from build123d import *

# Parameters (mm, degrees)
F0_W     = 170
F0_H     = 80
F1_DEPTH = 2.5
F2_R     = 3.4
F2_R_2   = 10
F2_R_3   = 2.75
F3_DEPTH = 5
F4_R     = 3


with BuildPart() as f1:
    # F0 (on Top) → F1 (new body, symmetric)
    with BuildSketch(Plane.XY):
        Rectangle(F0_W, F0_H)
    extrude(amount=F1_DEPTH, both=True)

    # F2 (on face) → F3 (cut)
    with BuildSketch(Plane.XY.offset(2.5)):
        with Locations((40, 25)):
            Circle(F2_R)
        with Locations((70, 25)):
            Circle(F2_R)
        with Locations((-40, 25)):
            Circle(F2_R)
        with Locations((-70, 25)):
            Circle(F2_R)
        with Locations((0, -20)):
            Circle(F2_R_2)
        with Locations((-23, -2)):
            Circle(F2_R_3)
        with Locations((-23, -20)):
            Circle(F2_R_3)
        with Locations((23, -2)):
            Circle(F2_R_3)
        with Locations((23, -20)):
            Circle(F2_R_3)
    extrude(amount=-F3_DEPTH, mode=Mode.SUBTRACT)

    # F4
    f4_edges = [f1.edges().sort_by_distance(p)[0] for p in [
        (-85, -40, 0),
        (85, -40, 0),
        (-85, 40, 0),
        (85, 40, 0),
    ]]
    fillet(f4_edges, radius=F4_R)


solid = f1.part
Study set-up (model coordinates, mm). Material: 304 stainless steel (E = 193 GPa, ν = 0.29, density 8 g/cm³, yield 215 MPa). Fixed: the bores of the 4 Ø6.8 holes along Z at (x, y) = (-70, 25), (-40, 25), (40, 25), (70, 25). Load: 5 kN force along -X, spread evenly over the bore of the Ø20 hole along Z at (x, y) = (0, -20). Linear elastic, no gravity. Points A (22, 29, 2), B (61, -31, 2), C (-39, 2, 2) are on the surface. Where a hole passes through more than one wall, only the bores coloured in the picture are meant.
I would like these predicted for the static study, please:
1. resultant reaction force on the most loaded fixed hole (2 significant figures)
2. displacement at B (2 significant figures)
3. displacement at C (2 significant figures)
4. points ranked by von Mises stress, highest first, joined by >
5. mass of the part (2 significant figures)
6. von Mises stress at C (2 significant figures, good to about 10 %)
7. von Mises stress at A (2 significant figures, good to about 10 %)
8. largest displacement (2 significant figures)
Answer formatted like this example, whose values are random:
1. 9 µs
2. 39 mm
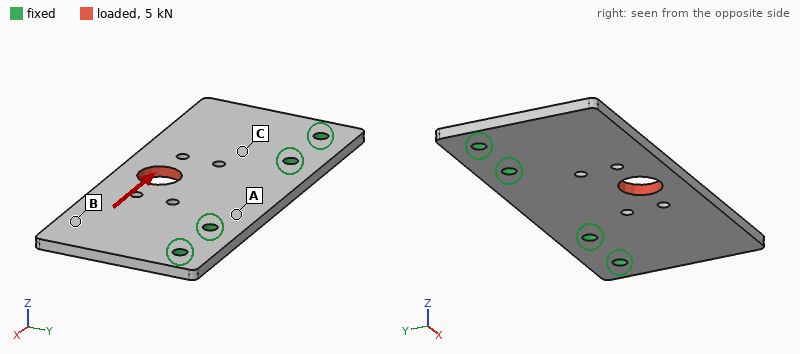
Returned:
1. 1.7 kN
2. 5.3 µm
3. 2.6 µm
4. C > A > B
5. 520 g
6. 11 MPa
7. 6.9 MPa
8. 8.1 µm
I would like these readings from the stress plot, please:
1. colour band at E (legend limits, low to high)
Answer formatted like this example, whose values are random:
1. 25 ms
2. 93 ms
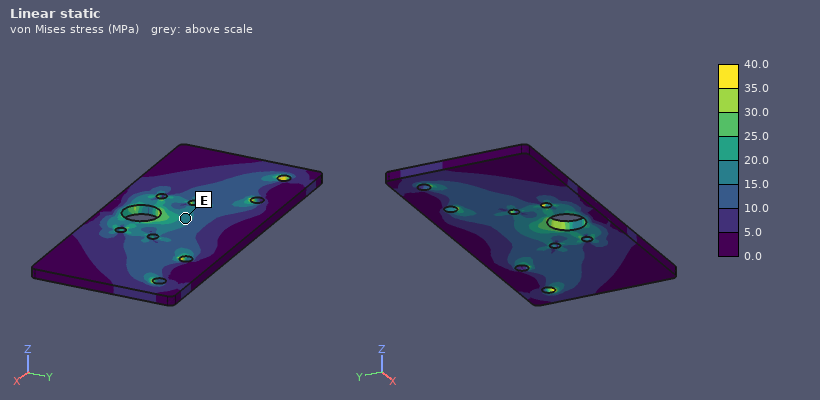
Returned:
1. 15.0 to 20.0 MPa
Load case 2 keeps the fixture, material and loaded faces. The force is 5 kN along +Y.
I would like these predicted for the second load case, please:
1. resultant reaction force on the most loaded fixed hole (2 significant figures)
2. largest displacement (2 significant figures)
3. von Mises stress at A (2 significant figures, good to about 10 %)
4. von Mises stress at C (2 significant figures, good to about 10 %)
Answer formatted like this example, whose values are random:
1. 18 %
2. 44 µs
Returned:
1. 2.4 kN
2. 9.0 µm
3. 9.4 MPa
4. 12 MPa
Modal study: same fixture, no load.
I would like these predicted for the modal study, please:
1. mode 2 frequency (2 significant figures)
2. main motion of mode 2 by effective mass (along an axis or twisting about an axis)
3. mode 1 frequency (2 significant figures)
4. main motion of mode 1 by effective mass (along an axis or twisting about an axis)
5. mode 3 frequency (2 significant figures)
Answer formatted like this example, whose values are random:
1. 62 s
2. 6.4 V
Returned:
1. 1300 Hz
2. twisting about Y
3. 900 Hz
4. along Z
5. 2000 Hz
